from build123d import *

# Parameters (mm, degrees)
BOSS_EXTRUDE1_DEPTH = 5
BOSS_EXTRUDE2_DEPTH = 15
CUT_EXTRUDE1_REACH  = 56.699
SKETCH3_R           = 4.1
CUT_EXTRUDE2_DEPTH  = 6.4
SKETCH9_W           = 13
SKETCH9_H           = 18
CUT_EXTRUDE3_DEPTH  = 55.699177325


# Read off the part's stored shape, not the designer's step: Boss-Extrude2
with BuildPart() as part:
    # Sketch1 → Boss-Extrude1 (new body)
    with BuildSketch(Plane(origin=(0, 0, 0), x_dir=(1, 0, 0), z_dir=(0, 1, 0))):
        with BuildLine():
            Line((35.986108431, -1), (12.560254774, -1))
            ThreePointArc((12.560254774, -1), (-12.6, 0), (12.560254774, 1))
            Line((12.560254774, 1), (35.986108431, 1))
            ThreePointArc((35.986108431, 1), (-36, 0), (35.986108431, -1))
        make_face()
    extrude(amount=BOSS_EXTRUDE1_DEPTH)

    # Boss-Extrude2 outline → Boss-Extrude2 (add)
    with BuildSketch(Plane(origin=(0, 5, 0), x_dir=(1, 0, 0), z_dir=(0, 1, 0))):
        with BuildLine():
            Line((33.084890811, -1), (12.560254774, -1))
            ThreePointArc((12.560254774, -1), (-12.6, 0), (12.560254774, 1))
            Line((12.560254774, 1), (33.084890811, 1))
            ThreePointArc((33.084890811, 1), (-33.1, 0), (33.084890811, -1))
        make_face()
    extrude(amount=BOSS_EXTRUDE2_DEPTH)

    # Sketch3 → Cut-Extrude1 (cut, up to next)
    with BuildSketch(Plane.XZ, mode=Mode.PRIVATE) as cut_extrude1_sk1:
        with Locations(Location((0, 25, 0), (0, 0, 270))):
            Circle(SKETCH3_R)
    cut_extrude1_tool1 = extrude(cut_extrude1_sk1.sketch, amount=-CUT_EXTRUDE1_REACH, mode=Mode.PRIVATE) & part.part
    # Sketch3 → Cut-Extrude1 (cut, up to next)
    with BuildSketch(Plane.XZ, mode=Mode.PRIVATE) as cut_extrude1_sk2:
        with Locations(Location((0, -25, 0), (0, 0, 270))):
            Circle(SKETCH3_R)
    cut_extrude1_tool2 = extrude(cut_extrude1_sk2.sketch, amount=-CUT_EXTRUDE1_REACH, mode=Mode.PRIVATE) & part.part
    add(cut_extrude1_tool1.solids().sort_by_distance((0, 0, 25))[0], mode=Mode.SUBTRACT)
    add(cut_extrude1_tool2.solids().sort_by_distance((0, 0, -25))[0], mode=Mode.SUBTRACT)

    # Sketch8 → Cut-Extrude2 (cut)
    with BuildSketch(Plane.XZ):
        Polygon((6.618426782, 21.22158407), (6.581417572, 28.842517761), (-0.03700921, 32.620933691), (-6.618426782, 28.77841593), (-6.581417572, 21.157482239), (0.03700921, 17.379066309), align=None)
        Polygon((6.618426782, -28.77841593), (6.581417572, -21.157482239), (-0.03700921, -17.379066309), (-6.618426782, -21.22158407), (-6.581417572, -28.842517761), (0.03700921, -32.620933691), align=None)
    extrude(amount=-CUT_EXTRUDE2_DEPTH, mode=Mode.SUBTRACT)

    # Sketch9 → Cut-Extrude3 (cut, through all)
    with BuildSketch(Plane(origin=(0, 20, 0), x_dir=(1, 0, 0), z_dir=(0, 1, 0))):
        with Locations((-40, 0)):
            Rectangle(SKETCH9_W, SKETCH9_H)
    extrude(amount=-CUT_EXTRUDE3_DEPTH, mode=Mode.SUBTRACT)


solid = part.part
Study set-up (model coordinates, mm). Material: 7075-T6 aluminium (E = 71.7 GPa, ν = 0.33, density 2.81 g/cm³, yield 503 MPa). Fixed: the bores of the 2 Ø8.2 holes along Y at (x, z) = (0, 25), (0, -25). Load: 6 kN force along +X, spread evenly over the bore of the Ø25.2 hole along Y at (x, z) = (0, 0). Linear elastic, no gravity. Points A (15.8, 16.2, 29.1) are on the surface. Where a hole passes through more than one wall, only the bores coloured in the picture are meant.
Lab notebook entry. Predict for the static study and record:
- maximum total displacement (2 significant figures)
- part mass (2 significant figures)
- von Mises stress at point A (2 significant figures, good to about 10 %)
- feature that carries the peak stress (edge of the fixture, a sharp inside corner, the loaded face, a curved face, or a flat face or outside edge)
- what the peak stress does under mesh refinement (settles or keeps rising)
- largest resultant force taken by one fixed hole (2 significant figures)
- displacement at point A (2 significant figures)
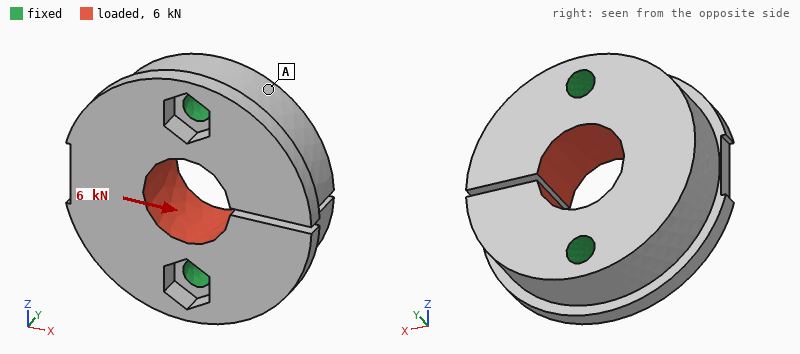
20 µm
160 g
6.3 MPa
edge of the fixture
keeps rising
3.3 kN
5.7 µm
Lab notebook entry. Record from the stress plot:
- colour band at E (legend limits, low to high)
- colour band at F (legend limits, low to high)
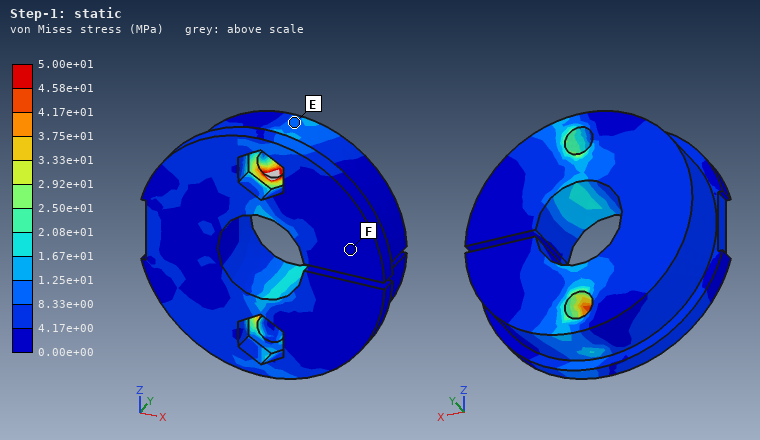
8.33e+00 to 1.25e+01 MPa
0.00e+00 to 4.17e+00 MPa
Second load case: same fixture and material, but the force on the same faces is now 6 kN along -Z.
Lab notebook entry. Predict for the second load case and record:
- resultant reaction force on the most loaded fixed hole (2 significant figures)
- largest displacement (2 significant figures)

3.0 kN
5.3 µm
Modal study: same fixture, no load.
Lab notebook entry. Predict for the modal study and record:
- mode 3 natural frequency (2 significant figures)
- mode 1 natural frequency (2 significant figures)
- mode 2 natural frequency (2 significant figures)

8800 Hz
7600 Hz
8300 Hz
